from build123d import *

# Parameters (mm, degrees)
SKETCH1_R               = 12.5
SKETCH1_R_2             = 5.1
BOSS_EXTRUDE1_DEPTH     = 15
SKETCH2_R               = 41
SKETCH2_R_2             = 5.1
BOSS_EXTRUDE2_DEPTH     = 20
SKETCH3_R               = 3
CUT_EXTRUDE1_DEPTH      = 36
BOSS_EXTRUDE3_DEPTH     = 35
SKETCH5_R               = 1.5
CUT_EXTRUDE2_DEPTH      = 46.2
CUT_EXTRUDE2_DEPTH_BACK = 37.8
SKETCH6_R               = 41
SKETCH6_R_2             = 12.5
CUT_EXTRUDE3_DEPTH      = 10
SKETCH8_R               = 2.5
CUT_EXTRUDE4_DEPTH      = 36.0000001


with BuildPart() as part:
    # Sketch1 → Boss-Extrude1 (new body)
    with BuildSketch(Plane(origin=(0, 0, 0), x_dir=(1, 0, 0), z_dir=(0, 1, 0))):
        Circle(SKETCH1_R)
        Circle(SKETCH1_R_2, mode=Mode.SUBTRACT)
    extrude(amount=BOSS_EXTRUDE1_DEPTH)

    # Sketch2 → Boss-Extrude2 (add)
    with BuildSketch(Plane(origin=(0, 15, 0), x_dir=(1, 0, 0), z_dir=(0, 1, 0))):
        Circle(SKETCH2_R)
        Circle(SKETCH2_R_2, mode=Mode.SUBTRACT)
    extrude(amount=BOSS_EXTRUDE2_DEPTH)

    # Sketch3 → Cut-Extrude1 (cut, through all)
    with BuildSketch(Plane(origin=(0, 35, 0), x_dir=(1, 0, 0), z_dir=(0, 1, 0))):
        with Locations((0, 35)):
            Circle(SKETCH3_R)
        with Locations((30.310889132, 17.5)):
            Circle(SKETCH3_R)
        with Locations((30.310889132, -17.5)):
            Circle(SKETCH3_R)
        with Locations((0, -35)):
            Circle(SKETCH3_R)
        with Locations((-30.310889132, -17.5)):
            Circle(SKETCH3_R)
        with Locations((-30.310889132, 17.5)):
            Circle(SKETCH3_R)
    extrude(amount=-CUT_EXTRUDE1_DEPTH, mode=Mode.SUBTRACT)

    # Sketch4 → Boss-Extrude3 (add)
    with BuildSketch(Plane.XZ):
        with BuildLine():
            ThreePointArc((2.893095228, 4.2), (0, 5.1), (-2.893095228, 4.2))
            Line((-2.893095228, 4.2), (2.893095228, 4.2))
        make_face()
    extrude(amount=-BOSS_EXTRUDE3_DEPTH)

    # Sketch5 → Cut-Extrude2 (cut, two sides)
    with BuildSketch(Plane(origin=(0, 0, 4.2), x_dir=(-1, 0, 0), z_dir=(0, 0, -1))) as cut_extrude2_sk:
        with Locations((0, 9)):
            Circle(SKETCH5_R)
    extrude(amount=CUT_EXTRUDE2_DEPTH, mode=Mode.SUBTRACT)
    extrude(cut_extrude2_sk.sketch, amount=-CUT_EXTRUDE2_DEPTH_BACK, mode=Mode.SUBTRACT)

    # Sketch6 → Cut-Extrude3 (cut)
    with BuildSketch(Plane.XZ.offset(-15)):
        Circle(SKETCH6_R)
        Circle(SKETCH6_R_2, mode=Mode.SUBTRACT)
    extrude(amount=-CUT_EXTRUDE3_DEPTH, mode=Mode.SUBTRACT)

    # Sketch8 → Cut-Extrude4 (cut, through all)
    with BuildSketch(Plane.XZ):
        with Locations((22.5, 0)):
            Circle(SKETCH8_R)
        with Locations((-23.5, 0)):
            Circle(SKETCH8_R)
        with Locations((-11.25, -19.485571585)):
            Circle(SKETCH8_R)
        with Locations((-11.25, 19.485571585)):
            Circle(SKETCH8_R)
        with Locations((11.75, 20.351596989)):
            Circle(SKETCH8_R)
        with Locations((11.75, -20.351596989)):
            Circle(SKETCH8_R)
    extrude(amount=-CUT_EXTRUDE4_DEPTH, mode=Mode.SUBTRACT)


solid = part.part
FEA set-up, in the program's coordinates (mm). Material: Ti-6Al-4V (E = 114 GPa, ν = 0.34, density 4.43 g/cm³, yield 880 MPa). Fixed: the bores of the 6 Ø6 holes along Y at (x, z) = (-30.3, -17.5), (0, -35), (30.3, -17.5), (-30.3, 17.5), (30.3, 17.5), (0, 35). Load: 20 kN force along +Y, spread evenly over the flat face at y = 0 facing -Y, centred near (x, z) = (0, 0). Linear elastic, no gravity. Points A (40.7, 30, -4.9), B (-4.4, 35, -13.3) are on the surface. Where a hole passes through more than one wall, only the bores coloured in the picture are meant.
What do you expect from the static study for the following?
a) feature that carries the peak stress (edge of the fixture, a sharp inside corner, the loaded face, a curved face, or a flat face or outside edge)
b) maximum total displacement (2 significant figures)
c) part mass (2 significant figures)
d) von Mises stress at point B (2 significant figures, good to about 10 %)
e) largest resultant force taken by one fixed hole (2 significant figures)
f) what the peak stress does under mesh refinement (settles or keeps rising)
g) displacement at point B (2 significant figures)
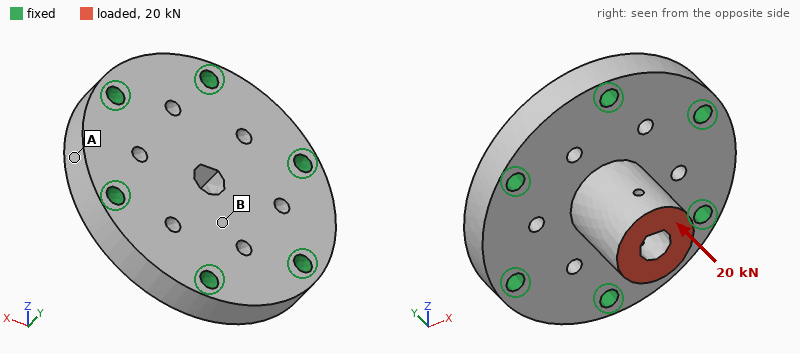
edge of the fixture
49 µm
260 g
72 MPa
3.5 kN
keeps rising
32 µm
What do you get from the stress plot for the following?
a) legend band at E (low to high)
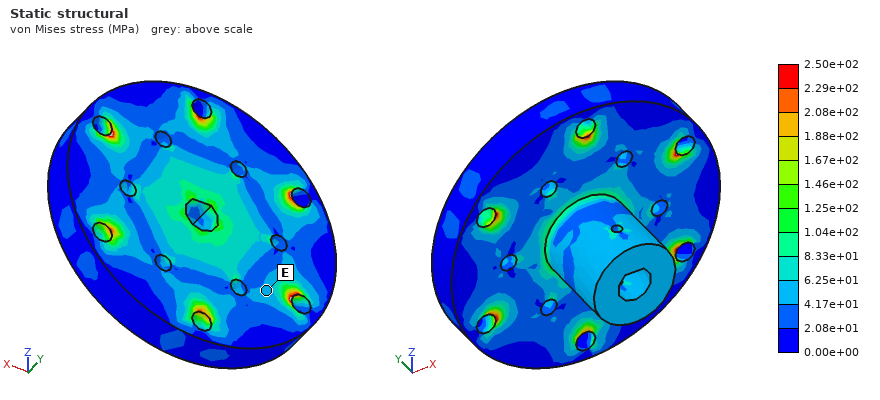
4.17e+01 to 6.25e+01 MPa
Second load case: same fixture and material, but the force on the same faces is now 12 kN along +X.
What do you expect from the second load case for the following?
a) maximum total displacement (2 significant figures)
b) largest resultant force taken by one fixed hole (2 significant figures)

0.14 mm
4.7 kN
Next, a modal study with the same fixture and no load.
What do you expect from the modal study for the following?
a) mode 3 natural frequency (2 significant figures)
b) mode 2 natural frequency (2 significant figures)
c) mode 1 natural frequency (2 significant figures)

12 kHz
11 kHz
11 kHz
